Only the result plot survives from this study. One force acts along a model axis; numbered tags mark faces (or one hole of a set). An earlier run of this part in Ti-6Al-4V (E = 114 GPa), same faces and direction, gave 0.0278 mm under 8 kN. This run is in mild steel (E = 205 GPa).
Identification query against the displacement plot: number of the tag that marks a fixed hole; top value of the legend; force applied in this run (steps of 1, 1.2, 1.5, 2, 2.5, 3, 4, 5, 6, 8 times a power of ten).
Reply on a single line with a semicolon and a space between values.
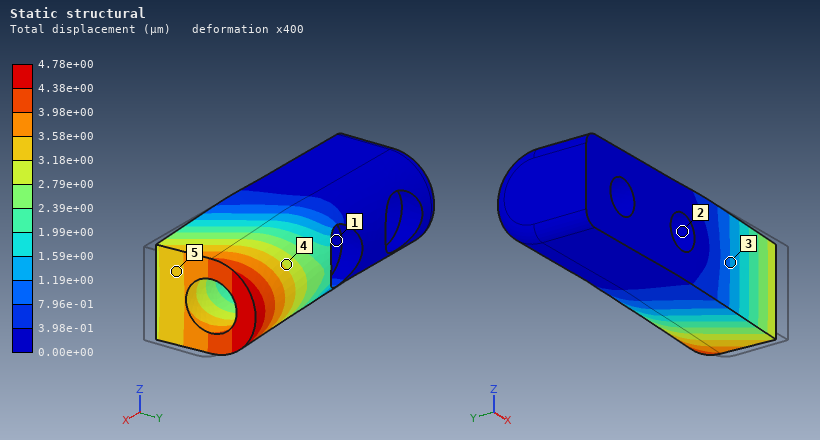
2; 4.78e+00 µm; 2.5 kN
